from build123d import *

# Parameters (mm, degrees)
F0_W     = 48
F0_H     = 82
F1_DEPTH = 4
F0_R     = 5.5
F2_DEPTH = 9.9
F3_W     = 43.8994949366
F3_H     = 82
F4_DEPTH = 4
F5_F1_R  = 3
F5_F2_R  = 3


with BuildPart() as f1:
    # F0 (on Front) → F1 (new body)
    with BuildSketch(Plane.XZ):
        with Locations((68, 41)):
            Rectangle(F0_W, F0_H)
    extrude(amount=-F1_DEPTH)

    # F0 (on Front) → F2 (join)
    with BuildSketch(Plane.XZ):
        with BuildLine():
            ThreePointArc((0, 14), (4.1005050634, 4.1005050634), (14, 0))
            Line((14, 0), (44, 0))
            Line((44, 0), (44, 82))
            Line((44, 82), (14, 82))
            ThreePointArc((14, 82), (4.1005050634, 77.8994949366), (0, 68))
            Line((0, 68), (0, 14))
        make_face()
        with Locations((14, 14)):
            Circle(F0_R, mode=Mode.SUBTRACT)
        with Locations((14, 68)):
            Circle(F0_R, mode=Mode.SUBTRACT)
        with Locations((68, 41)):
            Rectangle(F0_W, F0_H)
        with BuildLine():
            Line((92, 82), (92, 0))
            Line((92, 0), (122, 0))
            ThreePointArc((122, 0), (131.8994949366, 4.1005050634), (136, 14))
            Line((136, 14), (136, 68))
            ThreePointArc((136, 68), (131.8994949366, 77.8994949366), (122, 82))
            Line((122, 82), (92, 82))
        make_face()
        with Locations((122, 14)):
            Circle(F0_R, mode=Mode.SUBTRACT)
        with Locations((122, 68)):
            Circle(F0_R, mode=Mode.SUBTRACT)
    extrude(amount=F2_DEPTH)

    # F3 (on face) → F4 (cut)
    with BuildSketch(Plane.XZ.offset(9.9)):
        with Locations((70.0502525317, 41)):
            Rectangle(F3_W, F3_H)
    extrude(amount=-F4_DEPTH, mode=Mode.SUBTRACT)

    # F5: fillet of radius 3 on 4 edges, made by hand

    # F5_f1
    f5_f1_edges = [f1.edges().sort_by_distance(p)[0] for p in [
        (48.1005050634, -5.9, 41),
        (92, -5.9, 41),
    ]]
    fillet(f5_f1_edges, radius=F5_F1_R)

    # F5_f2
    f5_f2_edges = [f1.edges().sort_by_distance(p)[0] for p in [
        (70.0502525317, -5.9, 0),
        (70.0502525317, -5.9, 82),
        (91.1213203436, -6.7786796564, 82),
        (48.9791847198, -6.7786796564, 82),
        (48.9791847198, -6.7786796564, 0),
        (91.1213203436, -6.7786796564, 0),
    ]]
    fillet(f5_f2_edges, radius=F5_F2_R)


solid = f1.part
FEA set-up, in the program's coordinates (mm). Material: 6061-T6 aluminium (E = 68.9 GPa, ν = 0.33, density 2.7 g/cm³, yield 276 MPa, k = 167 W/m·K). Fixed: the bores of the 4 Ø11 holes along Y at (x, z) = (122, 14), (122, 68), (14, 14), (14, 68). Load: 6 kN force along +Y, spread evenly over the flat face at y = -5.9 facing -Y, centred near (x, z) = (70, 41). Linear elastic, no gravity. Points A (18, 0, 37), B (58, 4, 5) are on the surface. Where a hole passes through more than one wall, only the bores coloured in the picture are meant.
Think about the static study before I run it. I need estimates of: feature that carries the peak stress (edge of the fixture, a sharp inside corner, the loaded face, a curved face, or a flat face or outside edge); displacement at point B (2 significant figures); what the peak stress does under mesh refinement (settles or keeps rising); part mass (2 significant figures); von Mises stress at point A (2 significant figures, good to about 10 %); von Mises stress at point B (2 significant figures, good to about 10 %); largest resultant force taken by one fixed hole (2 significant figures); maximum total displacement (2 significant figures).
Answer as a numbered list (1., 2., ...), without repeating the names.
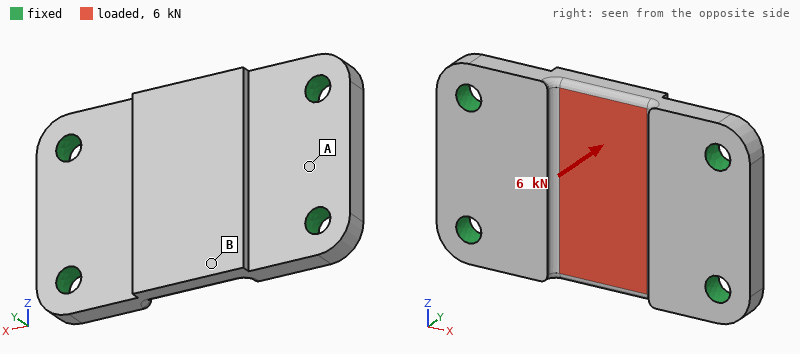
1. edge of the fixture
2. 55 µm
3. keeps rising
4. 290 g
5. 13 MPa
6. 29 MPa
7. 3.0 kN
8. 64 µm
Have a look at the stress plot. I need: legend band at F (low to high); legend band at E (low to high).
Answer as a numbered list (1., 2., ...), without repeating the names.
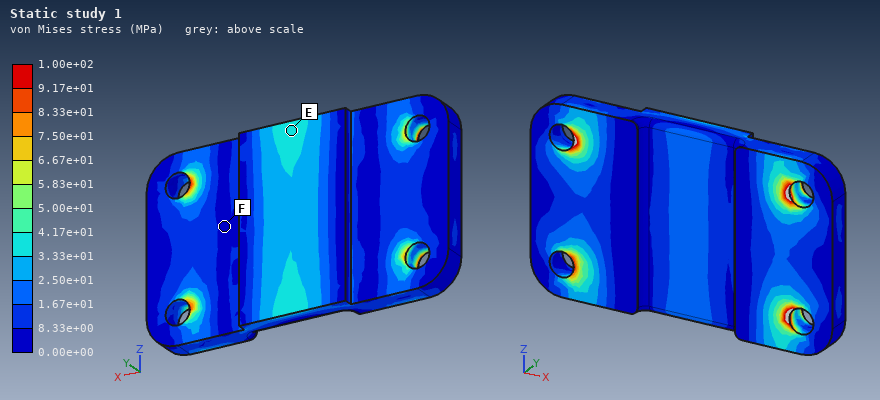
1. 0.00e+00 to 8.33e+00 MPa
2. 3.33e+01 to 4.17e+01 MPa
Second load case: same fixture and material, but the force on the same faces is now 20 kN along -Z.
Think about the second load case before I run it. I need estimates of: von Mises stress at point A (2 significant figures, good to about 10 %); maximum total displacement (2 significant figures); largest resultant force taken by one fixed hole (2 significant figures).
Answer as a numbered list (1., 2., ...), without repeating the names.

1. 14 MPa
2. 35 µm
3. 6.2 kN
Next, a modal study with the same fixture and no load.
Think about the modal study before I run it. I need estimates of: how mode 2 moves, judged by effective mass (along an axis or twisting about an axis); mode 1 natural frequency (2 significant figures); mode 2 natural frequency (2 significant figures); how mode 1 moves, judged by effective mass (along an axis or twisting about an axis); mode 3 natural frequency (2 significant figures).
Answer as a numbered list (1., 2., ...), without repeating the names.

1. twisting about X
2. 4700 Hz
3. 6000 Hz
4. along Y
5. 10 kHz
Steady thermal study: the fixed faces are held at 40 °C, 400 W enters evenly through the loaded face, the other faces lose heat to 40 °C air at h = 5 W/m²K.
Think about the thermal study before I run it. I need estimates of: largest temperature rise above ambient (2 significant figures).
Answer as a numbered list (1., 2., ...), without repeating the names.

1. 73 K
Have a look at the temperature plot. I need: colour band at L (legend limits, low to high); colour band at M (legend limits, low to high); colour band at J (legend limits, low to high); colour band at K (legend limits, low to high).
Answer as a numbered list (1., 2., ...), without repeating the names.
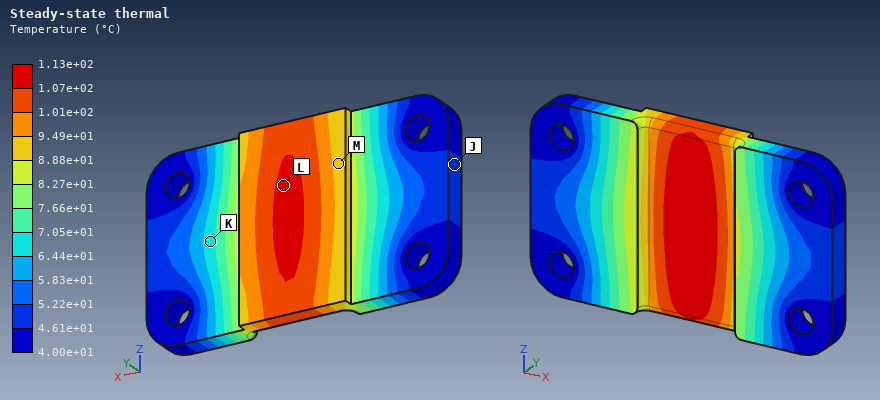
1. 1.07e+02 to 1.13e+02 °C
2. 8.88e+01 to 9.49e+01 °C
3. 4.61e+01 to 5.22e+01 °C
4. 6.44e+01 to 7.05e+01 °C
